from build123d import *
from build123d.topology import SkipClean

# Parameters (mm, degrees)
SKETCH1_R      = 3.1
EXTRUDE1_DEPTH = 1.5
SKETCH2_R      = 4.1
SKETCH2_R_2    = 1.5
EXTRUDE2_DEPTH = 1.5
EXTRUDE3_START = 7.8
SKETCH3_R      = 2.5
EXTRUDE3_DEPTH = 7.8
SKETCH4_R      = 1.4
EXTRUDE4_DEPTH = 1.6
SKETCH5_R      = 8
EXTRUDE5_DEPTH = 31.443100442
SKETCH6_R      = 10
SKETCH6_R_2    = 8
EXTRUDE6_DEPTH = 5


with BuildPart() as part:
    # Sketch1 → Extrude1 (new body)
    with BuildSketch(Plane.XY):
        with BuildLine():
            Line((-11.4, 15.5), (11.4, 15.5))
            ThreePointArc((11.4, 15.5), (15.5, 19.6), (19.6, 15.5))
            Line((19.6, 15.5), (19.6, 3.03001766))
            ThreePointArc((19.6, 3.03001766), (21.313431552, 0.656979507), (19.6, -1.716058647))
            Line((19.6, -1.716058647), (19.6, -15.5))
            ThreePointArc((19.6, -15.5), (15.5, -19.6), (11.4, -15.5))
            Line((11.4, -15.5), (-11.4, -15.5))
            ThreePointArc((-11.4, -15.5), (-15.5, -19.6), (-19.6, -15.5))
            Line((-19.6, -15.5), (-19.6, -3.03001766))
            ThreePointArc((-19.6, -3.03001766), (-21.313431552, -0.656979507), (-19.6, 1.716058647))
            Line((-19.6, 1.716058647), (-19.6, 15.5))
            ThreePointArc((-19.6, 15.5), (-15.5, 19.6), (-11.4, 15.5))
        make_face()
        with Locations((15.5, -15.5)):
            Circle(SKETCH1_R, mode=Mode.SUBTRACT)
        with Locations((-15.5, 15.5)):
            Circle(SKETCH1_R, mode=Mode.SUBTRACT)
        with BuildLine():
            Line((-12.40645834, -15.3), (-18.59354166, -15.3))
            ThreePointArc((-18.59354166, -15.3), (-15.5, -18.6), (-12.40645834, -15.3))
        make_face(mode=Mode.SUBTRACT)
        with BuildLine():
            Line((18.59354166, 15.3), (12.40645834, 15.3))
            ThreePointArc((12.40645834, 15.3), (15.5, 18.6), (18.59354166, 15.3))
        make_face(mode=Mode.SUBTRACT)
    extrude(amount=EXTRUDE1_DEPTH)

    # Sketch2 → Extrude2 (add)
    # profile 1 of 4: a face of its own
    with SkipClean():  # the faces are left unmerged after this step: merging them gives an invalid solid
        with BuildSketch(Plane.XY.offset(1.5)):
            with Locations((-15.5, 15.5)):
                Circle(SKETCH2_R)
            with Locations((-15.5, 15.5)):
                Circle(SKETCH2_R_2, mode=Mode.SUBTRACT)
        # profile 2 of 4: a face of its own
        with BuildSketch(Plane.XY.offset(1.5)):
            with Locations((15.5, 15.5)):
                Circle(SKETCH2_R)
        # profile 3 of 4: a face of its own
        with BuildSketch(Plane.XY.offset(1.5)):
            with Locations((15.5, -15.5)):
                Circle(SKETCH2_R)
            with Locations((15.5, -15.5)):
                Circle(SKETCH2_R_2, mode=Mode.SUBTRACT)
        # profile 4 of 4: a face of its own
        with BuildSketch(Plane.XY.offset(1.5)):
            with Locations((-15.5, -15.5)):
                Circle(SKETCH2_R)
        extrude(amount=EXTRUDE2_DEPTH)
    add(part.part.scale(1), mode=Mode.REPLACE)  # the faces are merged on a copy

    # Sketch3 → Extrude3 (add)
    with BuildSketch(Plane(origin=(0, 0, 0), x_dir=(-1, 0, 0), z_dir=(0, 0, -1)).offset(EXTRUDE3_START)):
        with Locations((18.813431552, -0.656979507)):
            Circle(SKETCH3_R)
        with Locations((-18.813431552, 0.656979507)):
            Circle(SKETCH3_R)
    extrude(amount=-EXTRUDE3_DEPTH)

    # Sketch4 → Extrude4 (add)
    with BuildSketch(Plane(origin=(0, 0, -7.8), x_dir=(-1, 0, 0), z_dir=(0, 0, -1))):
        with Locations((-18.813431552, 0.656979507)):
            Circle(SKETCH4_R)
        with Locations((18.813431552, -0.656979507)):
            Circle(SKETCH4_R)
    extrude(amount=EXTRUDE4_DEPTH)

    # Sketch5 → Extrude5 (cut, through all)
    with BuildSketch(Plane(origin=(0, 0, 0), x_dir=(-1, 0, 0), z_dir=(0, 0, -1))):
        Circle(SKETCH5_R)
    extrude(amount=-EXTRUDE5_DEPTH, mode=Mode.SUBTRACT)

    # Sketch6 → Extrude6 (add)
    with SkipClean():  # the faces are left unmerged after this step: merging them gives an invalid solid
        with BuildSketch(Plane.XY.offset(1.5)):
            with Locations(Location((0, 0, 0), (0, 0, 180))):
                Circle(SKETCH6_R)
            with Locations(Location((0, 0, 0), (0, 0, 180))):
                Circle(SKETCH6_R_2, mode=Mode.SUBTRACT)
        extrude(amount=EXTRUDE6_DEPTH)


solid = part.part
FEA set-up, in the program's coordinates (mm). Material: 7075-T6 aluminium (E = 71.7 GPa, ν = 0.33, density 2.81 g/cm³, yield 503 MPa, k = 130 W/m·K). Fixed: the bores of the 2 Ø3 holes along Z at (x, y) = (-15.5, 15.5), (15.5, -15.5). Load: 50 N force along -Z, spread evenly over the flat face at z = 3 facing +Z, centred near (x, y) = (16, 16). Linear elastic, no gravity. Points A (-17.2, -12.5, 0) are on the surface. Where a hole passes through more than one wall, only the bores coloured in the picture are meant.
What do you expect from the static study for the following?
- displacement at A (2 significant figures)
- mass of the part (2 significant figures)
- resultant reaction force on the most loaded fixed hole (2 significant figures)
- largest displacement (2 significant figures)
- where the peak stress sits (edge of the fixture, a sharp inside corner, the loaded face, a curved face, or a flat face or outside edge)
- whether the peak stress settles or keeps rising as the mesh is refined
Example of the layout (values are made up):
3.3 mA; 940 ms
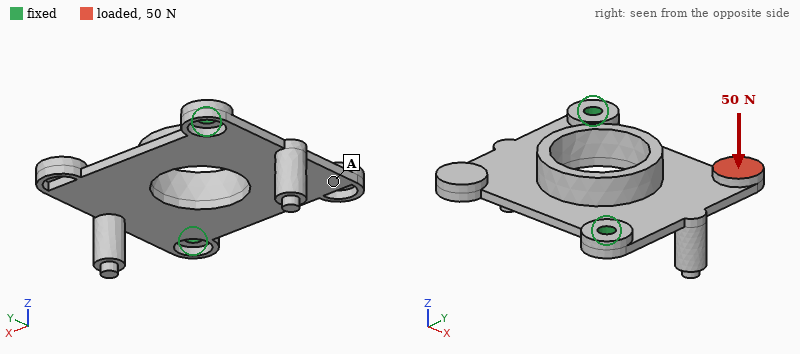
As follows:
0.19 mm; 7.7 g; 30 N; 0.50 mm; edge of the fixture; keeps rising
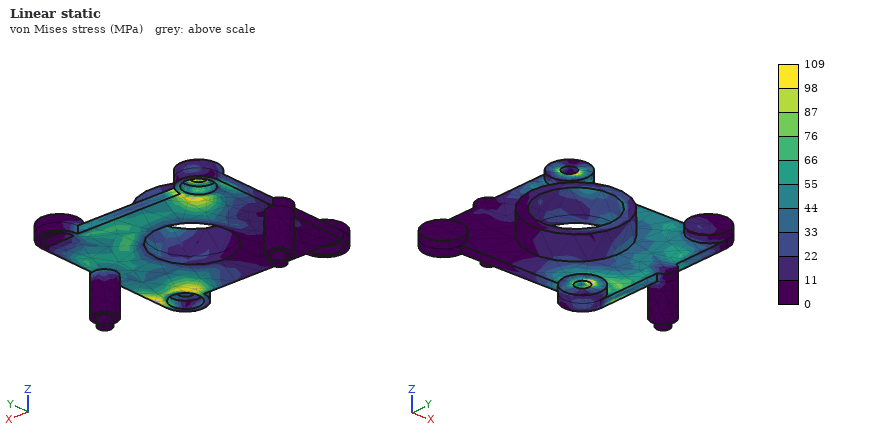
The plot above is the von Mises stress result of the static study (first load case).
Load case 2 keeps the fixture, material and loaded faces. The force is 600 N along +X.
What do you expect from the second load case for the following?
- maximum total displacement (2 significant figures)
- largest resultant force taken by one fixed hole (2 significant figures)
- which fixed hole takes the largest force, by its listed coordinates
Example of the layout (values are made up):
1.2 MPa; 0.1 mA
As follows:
0.52 mm; 500 N; (-15.5, 15.5)
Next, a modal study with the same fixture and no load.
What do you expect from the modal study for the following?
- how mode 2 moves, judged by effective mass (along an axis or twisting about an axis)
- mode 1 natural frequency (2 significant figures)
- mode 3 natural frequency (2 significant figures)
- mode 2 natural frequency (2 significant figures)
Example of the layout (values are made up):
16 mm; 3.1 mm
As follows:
along Z; 1500 Hz; 5900 Hz; 2600 Hz
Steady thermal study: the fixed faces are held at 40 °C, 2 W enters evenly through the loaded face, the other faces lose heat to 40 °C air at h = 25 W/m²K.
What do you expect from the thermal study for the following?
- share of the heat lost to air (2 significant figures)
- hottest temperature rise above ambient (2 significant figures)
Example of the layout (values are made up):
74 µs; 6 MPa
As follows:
19 %; 15 K
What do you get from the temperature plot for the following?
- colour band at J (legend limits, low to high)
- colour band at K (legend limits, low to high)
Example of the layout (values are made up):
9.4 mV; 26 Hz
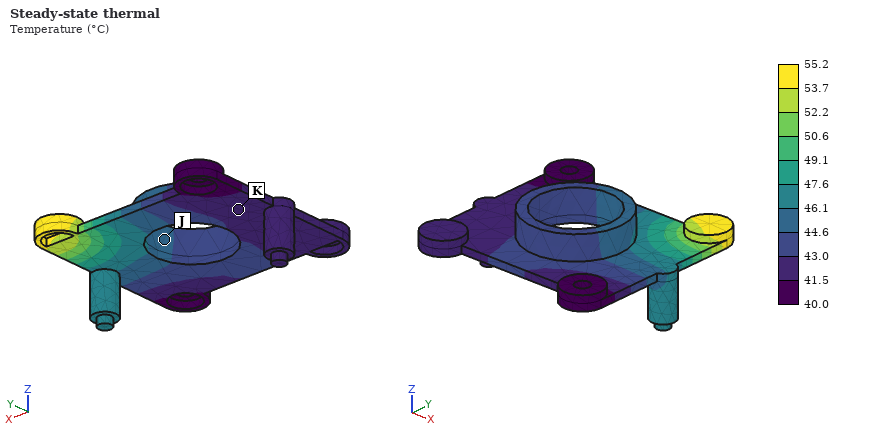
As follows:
44.6 to 46.1 °C; 41.5 to 43.0 °C
